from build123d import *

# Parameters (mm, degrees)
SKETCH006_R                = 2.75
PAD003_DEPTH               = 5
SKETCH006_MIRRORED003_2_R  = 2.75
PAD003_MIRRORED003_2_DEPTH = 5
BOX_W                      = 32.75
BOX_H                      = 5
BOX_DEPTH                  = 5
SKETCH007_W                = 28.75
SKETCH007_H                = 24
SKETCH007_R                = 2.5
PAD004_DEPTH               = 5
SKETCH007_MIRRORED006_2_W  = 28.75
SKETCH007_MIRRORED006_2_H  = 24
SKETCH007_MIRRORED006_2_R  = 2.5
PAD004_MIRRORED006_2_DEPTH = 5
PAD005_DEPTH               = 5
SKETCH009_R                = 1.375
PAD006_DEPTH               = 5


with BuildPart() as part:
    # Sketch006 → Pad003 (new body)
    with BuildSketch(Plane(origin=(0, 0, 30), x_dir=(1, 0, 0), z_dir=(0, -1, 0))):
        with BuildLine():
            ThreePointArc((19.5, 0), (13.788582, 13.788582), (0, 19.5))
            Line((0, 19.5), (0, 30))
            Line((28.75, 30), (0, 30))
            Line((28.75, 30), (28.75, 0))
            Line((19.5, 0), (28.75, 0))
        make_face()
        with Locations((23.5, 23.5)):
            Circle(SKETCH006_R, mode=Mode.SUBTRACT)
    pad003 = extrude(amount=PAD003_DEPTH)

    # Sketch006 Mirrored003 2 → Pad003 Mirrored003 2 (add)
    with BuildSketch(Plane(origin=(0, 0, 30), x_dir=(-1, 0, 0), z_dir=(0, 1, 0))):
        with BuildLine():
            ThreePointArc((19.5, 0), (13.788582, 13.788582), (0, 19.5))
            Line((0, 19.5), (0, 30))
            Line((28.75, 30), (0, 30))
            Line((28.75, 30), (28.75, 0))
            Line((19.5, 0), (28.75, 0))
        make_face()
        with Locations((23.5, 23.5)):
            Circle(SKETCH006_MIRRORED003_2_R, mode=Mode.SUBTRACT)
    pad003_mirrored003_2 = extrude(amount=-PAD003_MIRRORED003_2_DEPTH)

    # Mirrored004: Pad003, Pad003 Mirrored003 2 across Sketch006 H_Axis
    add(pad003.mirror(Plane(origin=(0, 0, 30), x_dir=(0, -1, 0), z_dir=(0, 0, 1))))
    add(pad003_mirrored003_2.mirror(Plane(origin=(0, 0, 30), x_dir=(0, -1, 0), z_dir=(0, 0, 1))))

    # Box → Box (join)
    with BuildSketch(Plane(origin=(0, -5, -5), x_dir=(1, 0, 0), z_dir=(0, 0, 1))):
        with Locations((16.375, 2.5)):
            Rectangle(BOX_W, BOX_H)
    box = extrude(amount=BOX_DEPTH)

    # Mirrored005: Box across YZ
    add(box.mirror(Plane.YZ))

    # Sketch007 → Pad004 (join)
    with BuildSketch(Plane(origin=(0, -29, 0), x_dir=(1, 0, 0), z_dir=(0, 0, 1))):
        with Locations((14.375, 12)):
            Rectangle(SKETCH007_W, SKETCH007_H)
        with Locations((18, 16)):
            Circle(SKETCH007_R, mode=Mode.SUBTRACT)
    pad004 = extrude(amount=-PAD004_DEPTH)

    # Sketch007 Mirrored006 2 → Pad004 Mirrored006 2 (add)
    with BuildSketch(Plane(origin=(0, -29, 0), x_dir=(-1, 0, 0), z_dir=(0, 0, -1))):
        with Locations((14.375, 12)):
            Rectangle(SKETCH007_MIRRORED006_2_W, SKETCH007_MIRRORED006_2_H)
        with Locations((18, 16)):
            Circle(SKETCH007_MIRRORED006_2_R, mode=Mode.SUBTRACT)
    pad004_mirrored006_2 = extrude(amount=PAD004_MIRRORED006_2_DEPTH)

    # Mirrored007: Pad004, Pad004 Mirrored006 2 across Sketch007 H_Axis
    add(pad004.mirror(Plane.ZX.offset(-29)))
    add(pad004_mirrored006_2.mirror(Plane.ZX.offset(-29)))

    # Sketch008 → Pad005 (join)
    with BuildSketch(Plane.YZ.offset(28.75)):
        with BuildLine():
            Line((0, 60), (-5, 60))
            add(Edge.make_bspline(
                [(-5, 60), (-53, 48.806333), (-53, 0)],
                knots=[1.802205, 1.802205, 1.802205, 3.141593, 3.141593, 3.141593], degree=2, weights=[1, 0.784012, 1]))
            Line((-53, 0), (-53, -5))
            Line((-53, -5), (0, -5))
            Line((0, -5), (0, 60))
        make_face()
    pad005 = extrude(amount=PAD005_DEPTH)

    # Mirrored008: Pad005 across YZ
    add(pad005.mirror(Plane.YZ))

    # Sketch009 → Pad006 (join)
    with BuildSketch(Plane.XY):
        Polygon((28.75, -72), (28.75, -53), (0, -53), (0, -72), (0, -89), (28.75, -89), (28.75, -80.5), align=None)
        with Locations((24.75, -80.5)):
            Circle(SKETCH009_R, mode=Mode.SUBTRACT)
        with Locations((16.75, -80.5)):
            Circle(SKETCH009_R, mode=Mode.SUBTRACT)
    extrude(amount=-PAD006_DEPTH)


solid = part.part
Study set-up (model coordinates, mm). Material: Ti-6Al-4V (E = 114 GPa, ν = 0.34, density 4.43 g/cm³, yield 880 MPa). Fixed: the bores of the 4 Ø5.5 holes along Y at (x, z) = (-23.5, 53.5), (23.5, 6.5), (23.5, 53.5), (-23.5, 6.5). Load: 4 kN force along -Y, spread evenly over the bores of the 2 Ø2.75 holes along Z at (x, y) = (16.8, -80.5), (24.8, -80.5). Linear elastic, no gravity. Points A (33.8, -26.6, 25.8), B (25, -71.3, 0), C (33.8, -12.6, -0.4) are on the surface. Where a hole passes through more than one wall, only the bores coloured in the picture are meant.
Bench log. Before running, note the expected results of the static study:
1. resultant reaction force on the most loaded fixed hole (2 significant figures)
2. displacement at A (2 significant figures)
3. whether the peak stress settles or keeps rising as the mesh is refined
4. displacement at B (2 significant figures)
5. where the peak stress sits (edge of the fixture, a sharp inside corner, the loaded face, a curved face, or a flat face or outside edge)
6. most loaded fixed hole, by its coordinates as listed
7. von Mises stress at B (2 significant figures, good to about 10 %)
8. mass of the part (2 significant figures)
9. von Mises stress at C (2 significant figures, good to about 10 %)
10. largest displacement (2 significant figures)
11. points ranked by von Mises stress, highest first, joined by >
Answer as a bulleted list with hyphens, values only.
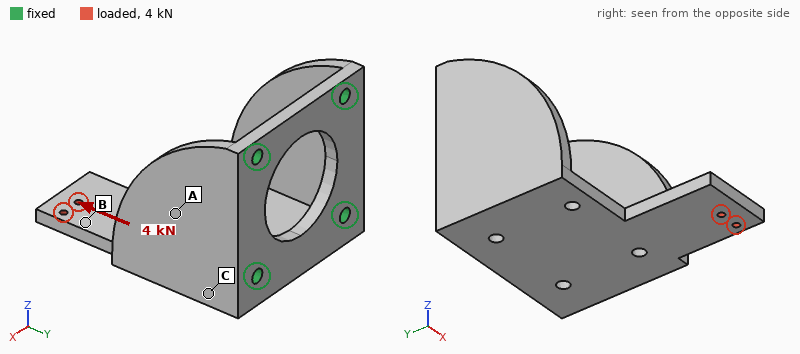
- 4.0 kN
- 12 µm
- keeps rising
- 55 µm
- edge of the fixture
- (23.5, 6.5)
- 54 MPa
- 260 g
- 18 MPa
- 77 µm
- B > C > A
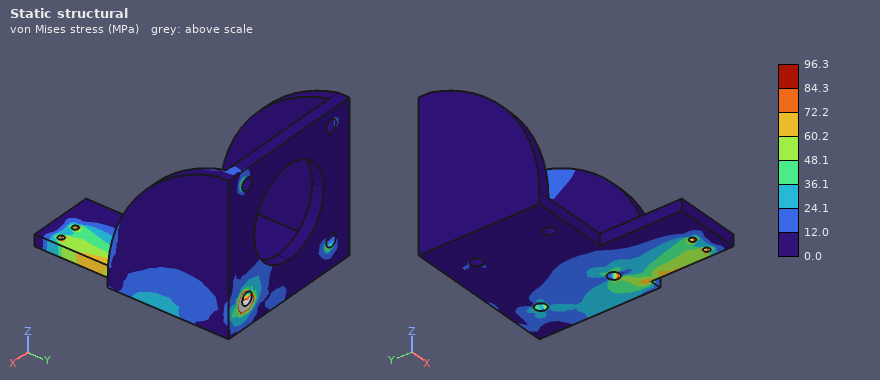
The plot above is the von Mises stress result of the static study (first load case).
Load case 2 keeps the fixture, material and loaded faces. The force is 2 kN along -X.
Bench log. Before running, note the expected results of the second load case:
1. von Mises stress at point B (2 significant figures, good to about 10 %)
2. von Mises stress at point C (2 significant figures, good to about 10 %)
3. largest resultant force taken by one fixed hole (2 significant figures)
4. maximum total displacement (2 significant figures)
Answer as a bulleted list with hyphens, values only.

- 29 MPa
- 16 MPa
- 3.5 kN
- 0.12 mm
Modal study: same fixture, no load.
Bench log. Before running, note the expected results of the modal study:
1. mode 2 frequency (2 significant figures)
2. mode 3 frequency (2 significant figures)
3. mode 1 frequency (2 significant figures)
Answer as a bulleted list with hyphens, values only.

- 3600 Hz
- 3600 Hz
- 1700 Hz
